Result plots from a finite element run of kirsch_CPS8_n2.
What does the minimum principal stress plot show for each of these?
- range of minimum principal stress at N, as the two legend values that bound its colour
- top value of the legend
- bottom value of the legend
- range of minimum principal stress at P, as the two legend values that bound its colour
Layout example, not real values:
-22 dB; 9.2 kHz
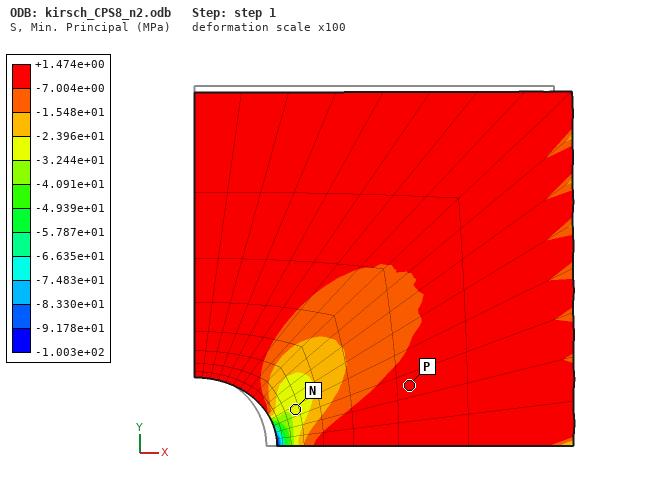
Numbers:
-3.244e+01 to -2.396e+01 MPa; +1.474e+00 MPa; -1.003e+02 MPa; -7.004e+00 to +1.474e+00 MPa
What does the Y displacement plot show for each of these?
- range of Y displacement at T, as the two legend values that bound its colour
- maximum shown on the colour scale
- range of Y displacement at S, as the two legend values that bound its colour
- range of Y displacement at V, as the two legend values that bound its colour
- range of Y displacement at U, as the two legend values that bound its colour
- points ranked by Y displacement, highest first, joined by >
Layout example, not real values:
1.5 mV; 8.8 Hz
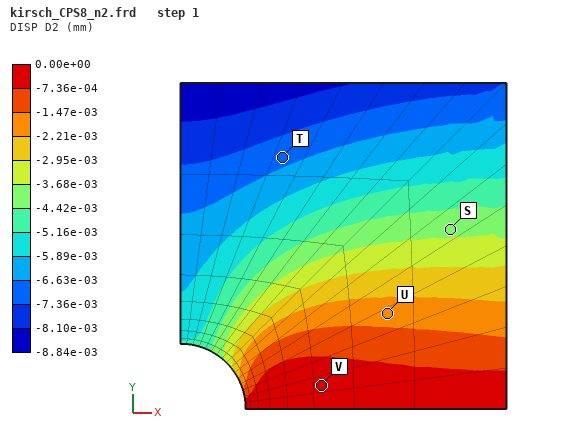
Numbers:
-7.36e-03 to -6.63e-03 mm; 0.00e+00 mm; -4.42e-03 to -3.68e-03 mm; -7.36e-04 to 0.00e+00 mm; -2.21e-03 to -1.47e-03 mm; V > U > S > T
